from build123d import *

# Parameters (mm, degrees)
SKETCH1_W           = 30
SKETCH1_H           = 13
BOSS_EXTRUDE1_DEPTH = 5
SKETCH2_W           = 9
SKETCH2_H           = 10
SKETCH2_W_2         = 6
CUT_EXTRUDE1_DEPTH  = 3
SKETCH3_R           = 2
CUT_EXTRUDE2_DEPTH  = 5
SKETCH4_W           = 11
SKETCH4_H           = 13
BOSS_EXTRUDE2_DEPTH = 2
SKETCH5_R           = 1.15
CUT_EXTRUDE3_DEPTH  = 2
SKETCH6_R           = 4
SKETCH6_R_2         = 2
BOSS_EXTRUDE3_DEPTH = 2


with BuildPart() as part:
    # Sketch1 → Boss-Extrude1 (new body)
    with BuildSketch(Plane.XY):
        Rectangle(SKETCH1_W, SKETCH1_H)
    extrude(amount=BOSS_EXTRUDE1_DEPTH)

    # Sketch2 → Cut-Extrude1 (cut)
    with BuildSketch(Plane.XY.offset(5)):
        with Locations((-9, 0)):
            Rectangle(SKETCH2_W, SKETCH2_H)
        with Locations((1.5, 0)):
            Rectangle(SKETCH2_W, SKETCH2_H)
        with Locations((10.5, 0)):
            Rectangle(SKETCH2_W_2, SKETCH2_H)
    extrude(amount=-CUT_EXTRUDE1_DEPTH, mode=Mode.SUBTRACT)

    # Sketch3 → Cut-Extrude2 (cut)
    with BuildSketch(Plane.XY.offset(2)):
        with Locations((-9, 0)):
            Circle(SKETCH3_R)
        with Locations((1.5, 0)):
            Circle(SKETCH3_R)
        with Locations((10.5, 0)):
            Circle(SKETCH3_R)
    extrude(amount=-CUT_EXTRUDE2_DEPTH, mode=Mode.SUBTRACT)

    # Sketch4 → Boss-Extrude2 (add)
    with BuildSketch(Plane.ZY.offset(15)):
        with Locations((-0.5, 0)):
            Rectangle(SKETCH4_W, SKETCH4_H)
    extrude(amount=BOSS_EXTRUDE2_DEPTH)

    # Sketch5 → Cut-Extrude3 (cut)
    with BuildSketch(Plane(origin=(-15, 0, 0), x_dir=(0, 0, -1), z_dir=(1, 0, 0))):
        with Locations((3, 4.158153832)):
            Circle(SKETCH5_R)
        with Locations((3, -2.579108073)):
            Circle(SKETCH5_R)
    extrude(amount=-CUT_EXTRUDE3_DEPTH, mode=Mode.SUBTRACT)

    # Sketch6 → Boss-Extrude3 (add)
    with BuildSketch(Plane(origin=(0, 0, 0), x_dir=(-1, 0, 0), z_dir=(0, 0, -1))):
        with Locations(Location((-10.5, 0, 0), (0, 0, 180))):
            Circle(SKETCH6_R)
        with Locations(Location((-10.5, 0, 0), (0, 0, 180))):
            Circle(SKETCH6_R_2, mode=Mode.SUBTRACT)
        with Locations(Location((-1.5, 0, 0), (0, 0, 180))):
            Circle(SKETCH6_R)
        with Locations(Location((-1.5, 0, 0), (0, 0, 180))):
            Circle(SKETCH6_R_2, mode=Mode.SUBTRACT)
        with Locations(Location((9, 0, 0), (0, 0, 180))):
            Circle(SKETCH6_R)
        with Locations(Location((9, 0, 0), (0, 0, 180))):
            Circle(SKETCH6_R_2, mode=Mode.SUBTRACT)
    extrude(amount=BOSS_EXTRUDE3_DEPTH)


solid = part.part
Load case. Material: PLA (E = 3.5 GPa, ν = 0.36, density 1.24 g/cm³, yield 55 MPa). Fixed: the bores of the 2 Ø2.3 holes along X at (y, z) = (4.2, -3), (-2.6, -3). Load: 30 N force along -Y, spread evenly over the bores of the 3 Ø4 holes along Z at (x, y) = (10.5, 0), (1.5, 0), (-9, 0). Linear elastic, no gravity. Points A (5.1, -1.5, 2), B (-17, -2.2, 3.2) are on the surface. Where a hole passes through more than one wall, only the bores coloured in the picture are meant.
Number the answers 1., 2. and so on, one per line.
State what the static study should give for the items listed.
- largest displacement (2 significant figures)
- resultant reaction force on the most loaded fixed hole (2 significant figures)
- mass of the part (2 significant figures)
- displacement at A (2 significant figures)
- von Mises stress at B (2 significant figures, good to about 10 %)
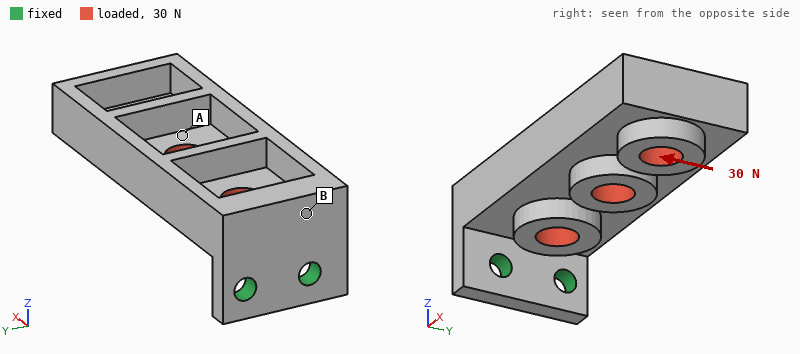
1. 0.39 mm
2. 62 N
3. 2.0 g
4. 0.25 mm
5. 6.4 MPa
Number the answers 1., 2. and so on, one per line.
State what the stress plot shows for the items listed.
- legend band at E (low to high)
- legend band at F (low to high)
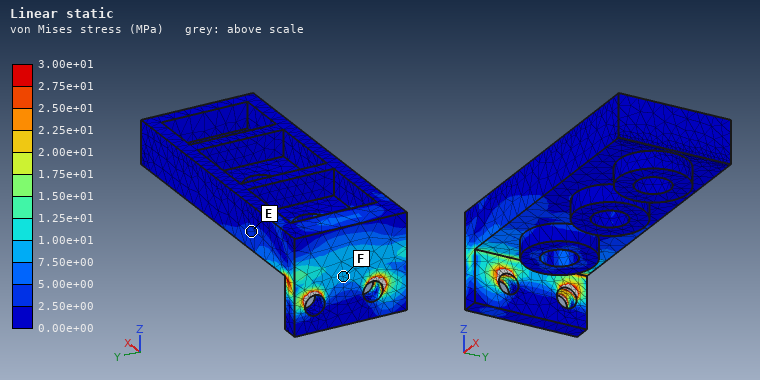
1. 2.50e+00 to 5.00e+00 MPa
2. 7.50e+00 to 1.00e+01 MPa
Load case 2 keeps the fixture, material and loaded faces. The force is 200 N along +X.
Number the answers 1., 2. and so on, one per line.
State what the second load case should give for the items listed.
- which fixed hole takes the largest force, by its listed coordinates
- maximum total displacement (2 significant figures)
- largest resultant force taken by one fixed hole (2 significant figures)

1. (-2.6, -3)
2. 0.19 mm
3. 120 N
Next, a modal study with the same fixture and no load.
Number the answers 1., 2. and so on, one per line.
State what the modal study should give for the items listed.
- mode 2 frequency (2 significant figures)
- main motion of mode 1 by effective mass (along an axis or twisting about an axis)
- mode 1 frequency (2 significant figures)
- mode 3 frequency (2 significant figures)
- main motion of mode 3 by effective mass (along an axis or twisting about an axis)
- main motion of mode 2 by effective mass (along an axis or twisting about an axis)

1. 1300 Hz
2. along Z
3. 550 Hz
4. 2700 Hz
5. twisting about X
6. along Y
